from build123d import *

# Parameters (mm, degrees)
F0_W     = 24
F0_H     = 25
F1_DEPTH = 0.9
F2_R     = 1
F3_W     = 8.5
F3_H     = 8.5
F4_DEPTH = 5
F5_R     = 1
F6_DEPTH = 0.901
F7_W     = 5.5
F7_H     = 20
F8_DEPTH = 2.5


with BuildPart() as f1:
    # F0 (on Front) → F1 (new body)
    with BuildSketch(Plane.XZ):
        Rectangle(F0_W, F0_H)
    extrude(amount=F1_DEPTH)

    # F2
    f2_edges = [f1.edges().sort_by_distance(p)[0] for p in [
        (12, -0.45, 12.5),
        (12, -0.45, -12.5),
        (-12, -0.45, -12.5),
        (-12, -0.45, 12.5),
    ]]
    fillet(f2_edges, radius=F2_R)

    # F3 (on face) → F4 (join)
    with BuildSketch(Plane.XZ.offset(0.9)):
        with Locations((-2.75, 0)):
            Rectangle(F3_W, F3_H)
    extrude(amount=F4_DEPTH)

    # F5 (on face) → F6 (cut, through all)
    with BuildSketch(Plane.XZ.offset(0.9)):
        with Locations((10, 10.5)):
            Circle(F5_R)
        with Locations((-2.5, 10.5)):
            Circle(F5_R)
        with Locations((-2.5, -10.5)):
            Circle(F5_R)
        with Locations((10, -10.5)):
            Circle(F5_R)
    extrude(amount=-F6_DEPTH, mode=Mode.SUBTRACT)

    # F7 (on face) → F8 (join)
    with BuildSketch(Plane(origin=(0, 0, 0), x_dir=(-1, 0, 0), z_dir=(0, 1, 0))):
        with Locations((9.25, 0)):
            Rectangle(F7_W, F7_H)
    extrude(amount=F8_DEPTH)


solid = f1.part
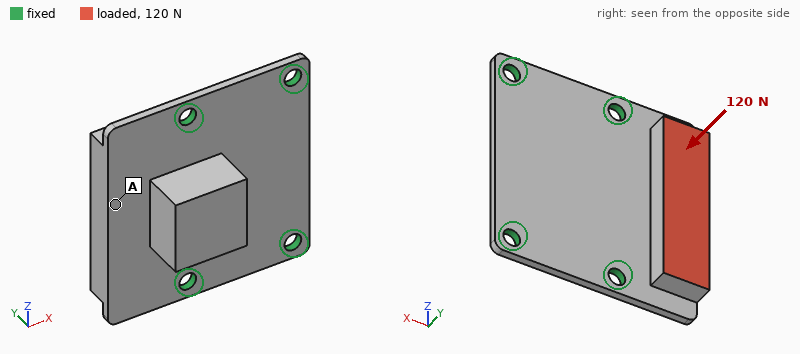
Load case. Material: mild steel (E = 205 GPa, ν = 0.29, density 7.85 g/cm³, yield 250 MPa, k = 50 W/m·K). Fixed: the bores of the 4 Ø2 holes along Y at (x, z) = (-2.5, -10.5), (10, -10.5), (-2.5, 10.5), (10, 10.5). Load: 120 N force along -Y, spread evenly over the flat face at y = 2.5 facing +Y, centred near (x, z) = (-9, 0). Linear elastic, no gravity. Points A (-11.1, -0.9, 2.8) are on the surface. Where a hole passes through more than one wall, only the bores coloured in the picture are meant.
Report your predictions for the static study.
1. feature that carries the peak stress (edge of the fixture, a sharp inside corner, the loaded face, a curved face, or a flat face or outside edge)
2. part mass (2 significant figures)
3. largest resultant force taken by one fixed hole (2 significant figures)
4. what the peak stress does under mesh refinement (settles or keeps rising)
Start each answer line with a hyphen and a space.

- edge of the fixture
- 9.1 g
- 75 N
- keeps rising
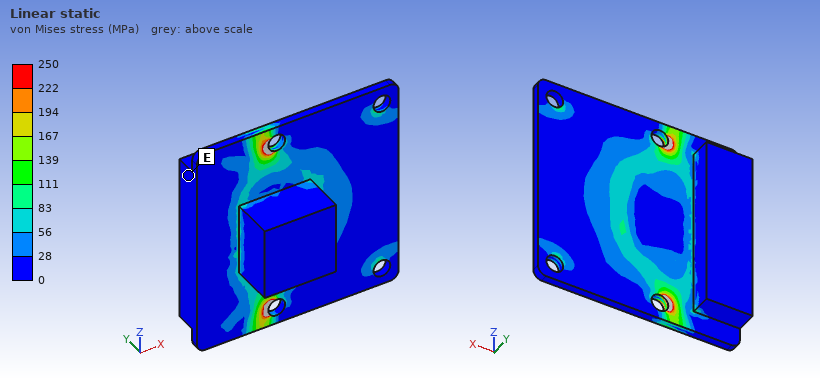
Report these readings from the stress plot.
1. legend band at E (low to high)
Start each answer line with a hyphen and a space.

- 0 to 28 MPa
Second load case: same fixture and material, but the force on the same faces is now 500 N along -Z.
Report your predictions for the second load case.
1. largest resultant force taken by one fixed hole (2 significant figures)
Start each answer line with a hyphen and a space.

- 280 N
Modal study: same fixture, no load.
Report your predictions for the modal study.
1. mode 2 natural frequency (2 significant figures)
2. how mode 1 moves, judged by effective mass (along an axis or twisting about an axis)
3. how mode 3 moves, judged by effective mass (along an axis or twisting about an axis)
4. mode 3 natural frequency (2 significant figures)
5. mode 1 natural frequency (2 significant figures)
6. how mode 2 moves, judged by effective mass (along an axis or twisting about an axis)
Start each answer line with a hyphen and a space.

- 9800 Hz
- along Y
- twisting about X
- 16 kHz
- 5200 Hz
- along Y
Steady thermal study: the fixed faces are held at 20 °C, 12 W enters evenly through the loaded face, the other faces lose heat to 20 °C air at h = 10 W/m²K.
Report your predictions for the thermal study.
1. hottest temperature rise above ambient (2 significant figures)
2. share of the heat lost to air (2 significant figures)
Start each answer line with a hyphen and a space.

- 78 K
- 4.3 %
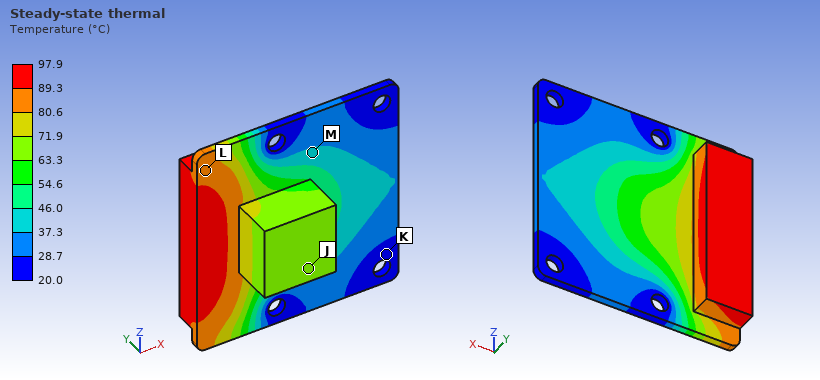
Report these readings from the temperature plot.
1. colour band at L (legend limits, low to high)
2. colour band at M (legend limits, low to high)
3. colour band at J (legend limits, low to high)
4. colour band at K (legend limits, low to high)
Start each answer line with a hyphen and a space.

- 80.6 to 89.3 °C
- 37.3 to 46.0 °C
- 63.3 to 71.9 °C
- 20.0 to 28.7 °C
